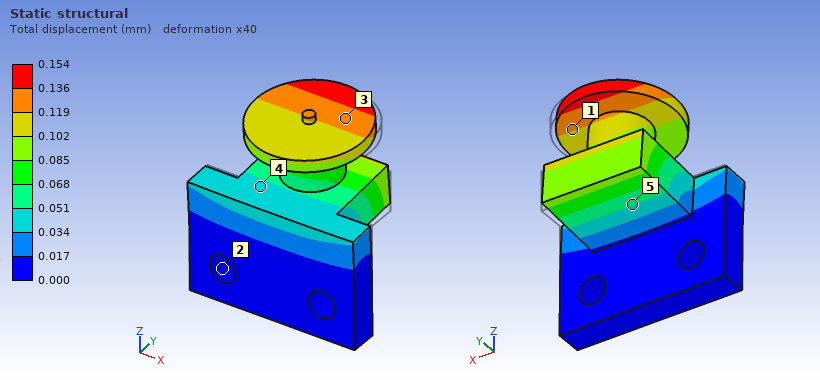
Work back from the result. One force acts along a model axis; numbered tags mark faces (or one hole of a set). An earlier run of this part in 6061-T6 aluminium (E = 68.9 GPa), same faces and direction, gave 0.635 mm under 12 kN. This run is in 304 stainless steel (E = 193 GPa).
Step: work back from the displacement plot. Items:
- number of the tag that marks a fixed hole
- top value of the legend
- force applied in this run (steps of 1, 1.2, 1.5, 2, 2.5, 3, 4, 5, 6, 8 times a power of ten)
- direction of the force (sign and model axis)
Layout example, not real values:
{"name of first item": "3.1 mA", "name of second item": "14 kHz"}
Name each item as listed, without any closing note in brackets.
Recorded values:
{"number of the tag that marks a fixed hole": "2", "top value of the legend": "0.154 mm", "force applied in this run": "8 kN", "direction of the force": "+Z"}
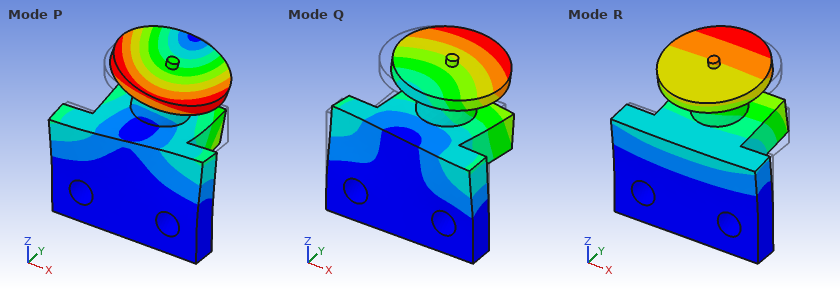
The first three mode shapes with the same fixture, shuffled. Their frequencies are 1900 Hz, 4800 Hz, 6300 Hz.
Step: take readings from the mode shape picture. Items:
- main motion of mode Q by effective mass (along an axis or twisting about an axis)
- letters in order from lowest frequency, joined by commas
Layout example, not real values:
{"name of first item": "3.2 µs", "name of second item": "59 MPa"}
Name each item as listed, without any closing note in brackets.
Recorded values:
{"main motion of mode Q by effective mass": "along X", "letters in order from lowest frequency, joined by commas": "R, Q, P"}
